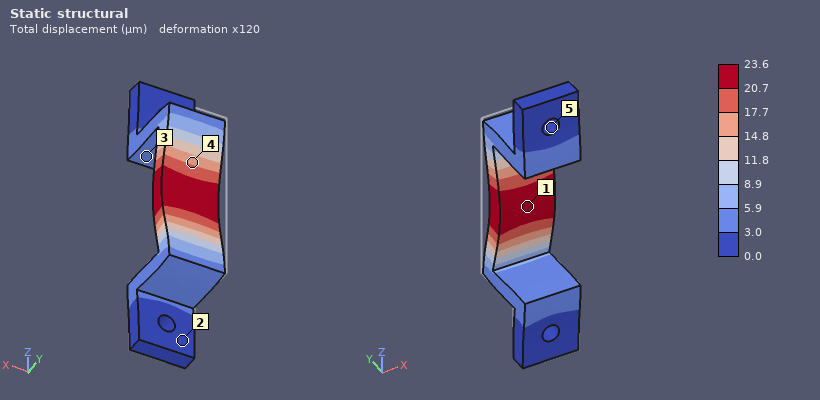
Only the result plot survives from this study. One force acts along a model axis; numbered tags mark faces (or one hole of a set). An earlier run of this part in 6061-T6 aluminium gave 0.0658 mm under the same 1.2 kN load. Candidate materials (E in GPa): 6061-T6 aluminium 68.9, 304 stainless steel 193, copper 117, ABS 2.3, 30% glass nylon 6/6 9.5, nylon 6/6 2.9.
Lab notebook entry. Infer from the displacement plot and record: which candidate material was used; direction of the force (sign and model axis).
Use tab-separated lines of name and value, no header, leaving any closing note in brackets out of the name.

which candidate material was used	304 stainless steel
direction of the force	-Y
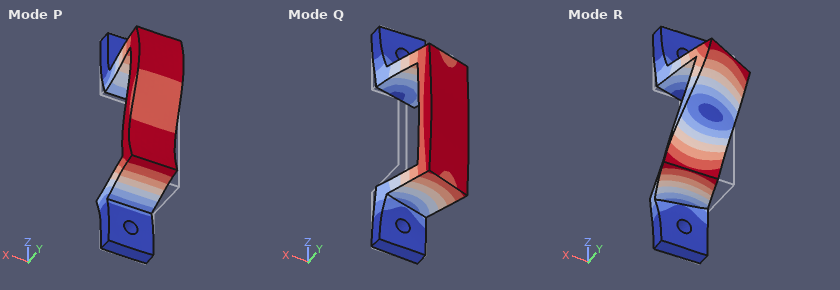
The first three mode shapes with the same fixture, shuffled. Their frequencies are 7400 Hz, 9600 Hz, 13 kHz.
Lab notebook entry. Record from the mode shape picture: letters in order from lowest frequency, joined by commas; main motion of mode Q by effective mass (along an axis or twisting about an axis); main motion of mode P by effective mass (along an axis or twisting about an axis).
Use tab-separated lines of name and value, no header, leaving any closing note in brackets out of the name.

letters in order from lowest frequency, joined by commas	Q, P, R
main motion of mode Q by effective mass	along X
main motion of mode P by effective mass	along Z
